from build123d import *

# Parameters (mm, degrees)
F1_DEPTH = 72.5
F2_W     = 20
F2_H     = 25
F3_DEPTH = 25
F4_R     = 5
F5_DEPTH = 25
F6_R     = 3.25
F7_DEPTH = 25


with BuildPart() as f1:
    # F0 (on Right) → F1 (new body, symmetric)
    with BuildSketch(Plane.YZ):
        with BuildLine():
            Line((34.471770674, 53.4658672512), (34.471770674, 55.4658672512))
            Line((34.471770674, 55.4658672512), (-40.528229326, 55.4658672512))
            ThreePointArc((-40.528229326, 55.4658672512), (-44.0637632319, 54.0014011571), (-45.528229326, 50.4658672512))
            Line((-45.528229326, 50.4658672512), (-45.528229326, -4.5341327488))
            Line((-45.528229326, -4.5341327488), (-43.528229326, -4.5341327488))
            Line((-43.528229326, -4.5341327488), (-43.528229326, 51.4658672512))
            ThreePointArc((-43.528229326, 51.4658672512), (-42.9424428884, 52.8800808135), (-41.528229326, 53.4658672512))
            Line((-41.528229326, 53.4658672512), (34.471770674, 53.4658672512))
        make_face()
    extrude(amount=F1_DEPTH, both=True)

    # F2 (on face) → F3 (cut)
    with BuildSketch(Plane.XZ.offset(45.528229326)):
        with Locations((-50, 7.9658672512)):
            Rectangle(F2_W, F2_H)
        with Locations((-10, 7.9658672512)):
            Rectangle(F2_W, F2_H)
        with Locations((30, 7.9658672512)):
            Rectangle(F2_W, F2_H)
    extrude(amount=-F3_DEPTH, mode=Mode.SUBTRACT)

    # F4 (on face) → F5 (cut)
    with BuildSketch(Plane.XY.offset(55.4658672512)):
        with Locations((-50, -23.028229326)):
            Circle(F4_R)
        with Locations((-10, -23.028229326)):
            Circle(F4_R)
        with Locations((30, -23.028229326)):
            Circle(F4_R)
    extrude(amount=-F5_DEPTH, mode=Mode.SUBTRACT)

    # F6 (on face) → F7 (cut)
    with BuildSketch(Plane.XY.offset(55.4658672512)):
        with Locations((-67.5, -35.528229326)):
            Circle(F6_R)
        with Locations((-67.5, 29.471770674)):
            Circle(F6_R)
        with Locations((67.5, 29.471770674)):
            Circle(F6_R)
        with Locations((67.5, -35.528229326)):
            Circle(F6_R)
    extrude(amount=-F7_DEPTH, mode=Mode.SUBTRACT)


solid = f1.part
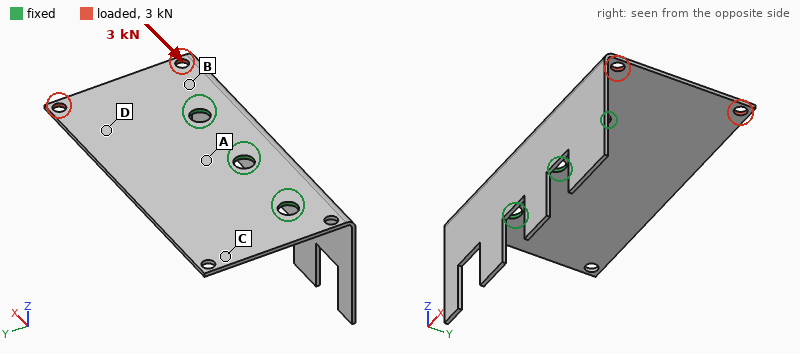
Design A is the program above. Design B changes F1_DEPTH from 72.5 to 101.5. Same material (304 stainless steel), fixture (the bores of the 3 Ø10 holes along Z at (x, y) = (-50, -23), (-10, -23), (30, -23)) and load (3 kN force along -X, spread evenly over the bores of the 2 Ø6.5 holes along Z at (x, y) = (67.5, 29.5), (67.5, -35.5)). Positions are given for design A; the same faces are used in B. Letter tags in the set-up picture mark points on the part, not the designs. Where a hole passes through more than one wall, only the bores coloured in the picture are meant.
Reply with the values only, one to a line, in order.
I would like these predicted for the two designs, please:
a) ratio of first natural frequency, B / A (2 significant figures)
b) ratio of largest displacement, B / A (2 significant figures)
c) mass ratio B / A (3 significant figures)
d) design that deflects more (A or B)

0.80
0.74
1.44
A
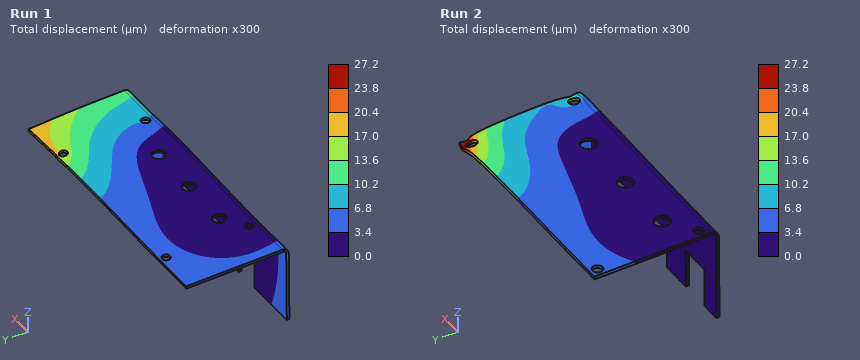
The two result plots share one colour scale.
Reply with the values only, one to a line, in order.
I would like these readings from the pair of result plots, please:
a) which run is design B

Run 1
